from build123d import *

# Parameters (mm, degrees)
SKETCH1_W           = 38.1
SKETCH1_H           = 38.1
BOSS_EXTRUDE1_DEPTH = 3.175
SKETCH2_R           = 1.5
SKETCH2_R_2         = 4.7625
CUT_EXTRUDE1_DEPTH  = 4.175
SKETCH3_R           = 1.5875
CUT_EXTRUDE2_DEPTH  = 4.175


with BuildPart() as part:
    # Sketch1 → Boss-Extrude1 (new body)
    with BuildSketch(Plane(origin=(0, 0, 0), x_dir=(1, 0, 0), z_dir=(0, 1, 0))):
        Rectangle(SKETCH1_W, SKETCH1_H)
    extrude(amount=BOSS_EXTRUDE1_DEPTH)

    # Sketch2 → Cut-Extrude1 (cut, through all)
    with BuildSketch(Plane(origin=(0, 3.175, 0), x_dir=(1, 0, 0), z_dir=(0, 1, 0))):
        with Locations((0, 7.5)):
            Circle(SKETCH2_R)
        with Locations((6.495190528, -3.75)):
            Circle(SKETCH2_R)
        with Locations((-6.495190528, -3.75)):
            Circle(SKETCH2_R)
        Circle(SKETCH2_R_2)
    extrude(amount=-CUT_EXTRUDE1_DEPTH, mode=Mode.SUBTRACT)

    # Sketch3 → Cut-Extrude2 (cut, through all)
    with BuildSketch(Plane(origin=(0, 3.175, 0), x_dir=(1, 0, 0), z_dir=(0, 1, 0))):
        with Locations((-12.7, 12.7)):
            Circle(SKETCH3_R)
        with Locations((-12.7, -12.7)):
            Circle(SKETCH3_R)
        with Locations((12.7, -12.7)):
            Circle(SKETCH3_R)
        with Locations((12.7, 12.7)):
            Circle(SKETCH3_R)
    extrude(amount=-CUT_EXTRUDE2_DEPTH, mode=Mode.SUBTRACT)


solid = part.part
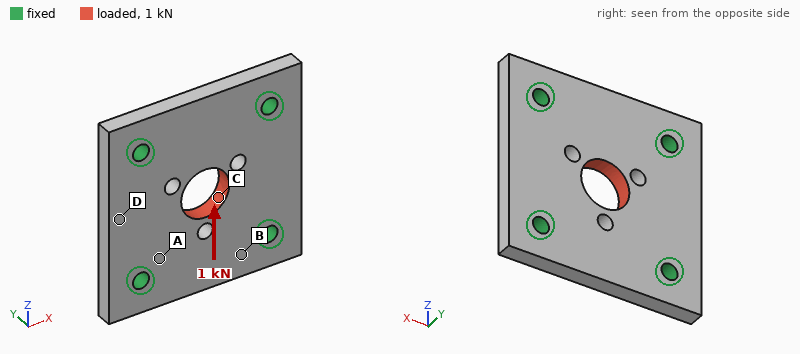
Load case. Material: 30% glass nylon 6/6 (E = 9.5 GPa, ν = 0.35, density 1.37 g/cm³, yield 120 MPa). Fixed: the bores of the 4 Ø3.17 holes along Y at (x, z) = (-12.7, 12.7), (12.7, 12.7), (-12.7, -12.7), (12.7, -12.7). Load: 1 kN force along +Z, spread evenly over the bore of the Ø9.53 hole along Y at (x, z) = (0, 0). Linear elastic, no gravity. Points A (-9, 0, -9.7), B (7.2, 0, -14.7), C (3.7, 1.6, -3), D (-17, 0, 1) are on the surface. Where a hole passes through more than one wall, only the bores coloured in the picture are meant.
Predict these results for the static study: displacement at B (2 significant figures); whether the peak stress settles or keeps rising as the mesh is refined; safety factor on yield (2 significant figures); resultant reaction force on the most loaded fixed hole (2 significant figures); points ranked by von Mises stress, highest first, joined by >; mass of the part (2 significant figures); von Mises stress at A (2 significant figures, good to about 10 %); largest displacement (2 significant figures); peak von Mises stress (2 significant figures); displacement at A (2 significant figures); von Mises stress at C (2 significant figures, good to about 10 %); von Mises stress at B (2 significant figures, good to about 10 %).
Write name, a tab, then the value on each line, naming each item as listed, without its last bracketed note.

displacement at B	8.3 µm
whether the peak stress settles or keeps rising as the mesh is refined	settles
safety factor on yield	3.7
resultant reaction force on the most loaded fixed hole	280 N
points ranked by von Mises stress, highest first, joined by >	C > A > B > D
mass of the part	5.8 g
von Mises stress at A	11 MPa
largest displacement	25 µm
peak von Mises stress	32 MPa
displacement at A	6.1 µm
von Mises stress at C	16 MPa
von Mises stress at B	6.0 MPa
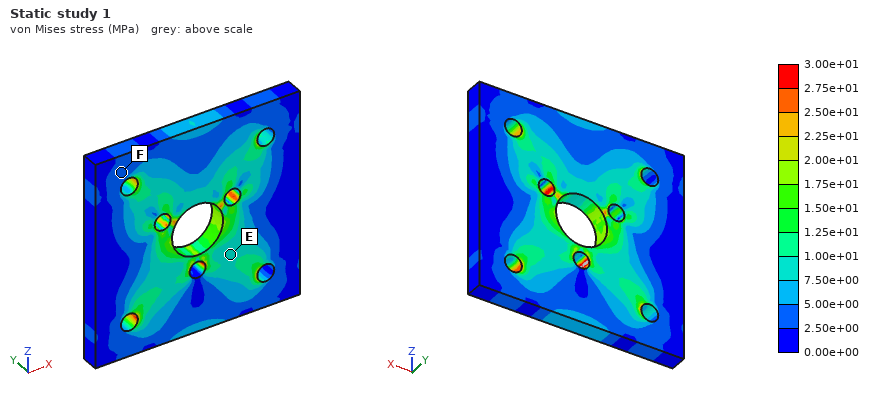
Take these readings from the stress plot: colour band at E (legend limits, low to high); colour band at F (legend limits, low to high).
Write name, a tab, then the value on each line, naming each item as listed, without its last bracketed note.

colour band at E	7.50e+00 to 1.00e+01 MPa
colour band at F	2.50e+00 to 5.00e+00 MPa
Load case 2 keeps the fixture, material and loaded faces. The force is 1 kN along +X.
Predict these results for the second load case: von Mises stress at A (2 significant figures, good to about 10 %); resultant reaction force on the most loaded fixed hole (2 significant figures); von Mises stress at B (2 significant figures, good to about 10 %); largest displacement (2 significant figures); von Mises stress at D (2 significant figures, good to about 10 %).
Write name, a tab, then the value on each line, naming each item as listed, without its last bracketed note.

von Mises stress at A	10 MPa
resultant reaction force on the most loaded fixed hole	280 N
von Mises stress at B	2.9 MPa
largest displacement	23 µm
von Mises stress at D	4.8 MPa
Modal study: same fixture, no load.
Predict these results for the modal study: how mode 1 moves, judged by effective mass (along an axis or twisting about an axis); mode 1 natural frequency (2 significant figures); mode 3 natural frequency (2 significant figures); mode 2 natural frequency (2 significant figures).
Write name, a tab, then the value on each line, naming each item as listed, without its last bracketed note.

how mode 1 moves, judged by effective mass	along Y
mode 1 natural frequency	10 kHz
mode 3 natural frequency	13 kHz
mode 2 natural frequency	13 kHz
